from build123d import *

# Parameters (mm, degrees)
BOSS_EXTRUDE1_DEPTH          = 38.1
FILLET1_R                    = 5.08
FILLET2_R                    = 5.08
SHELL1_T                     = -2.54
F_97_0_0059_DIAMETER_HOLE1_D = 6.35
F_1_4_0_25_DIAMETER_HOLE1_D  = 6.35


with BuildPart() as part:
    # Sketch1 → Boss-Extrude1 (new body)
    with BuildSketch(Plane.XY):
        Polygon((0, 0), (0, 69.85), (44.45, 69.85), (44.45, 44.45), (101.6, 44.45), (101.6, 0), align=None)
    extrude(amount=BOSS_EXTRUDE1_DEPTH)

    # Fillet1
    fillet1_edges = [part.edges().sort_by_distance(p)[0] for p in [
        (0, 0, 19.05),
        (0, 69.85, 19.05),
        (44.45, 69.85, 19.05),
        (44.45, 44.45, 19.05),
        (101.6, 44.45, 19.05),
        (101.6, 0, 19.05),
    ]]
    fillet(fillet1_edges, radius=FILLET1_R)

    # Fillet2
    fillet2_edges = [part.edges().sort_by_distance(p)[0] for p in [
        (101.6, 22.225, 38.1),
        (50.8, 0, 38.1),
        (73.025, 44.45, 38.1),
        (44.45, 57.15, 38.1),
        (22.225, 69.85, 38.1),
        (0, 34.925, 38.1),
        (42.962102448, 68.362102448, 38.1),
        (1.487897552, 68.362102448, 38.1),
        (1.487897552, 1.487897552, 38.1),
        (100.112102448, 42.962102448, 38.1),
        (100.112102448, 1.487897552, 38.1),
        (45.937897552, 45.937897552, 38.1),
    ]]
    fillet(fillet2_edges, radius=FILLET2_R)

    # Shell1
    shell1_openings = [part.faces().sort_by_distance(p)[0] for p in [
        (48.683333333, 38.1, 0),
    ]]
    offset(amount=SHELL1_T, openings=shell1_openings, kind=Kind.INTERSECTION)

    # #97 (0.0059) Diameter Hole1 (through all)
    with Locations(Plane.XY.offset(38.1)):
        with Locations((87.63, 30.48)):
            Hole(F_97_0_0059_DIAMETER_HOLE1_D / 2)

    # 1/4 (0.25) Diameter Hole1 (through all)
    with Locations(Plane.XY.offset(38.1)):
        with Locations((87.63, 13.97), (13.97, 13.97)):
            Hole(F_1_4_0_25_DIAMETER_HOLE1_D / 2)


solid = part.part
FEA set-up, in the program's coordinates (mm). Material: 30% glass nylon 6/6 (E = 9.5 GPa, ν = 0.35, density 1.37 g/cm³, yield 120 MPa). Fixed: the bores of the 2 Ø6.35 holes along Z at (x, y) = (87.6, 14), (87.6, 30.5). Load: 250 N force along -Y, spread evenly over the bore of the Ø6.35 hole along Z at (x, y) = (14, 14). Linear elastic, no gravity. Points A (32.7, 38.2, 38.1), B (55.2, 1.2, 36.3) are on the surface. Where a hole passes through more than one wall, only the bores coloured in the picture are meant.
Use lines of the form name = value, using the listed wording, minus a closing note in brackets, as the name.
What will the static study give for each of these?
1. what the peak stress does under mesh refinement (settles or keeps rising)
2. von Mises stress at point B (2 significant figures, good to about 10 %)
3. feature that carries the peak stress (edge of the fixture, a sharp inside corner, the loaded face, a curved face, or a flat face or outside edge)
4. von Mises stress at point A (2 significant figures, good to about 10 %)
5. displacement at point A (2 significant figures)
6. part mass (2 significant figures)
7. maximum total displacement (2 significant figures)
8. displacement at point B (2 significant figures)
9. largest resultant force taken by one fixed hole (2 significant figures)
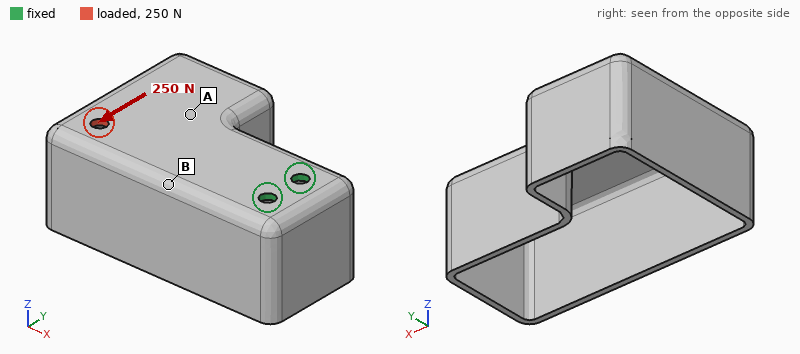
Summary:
what the peak stress does under mesh refinement = keeps rising
von Mises stress at point B = 6.7 MPa
feature that carries the peak stress = edge of the fixture
von Mises stress at point A = 3.1 MPa
displacement at point A = 0.21 mm
part mass = 57 g
maximum total displacement = 0.45 mm
displacement at point B = 0.13 mm
largest resultant force taken by one fixed hole = 850 N
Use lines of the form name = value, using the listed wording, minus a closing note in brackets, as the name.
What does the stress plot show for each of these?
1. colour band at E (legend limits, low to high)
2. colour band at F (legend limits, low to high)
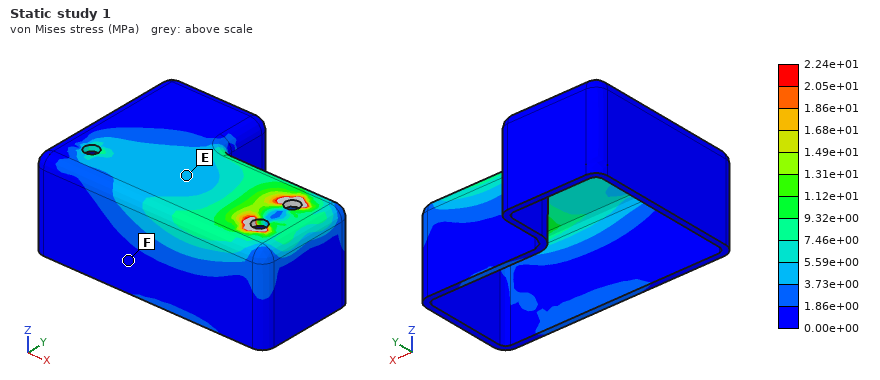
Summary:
colour band at E = 3.73e+00 to 5.59e+00 MPa
colour band at F = 0.00e+00 to 1.86e+00 MPa
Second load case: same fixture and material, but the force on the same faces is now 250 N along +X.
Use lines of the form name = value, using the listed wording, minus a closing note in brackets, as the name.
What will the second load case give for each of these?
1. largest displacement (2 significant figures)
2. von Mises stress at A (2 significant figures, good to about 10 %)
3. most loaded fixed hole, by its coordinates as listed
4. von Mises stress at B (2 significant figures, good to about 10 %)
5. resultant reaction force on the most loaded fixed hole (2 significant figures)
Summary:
largest displacement = 59 µm
von Mises stress at A = 0.79 MPa
most loaded fixed hole, by its coordinates as listed = (87.6, 14)
von Mises stress at B = 2.8 MPa
resultant reaction force on the most loaded fixed hole = 220 N
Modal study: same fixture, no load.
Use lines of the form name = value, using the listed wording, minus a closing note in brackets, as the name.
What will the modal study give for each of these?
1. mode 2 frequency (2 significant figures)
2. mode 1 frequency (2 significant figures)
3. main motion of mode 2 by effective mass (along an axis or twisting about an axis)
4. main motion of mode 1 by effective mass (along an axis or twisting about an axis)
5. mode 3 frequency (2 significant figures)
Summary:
mode 2 frequency = 280 Hz
mode 1 frequency = 170 Hz
main motion of mode 2 by effective mass = along Y
main motion of mode 1 by effective mass = along Z
mode 3 frequency = 770 Hz
